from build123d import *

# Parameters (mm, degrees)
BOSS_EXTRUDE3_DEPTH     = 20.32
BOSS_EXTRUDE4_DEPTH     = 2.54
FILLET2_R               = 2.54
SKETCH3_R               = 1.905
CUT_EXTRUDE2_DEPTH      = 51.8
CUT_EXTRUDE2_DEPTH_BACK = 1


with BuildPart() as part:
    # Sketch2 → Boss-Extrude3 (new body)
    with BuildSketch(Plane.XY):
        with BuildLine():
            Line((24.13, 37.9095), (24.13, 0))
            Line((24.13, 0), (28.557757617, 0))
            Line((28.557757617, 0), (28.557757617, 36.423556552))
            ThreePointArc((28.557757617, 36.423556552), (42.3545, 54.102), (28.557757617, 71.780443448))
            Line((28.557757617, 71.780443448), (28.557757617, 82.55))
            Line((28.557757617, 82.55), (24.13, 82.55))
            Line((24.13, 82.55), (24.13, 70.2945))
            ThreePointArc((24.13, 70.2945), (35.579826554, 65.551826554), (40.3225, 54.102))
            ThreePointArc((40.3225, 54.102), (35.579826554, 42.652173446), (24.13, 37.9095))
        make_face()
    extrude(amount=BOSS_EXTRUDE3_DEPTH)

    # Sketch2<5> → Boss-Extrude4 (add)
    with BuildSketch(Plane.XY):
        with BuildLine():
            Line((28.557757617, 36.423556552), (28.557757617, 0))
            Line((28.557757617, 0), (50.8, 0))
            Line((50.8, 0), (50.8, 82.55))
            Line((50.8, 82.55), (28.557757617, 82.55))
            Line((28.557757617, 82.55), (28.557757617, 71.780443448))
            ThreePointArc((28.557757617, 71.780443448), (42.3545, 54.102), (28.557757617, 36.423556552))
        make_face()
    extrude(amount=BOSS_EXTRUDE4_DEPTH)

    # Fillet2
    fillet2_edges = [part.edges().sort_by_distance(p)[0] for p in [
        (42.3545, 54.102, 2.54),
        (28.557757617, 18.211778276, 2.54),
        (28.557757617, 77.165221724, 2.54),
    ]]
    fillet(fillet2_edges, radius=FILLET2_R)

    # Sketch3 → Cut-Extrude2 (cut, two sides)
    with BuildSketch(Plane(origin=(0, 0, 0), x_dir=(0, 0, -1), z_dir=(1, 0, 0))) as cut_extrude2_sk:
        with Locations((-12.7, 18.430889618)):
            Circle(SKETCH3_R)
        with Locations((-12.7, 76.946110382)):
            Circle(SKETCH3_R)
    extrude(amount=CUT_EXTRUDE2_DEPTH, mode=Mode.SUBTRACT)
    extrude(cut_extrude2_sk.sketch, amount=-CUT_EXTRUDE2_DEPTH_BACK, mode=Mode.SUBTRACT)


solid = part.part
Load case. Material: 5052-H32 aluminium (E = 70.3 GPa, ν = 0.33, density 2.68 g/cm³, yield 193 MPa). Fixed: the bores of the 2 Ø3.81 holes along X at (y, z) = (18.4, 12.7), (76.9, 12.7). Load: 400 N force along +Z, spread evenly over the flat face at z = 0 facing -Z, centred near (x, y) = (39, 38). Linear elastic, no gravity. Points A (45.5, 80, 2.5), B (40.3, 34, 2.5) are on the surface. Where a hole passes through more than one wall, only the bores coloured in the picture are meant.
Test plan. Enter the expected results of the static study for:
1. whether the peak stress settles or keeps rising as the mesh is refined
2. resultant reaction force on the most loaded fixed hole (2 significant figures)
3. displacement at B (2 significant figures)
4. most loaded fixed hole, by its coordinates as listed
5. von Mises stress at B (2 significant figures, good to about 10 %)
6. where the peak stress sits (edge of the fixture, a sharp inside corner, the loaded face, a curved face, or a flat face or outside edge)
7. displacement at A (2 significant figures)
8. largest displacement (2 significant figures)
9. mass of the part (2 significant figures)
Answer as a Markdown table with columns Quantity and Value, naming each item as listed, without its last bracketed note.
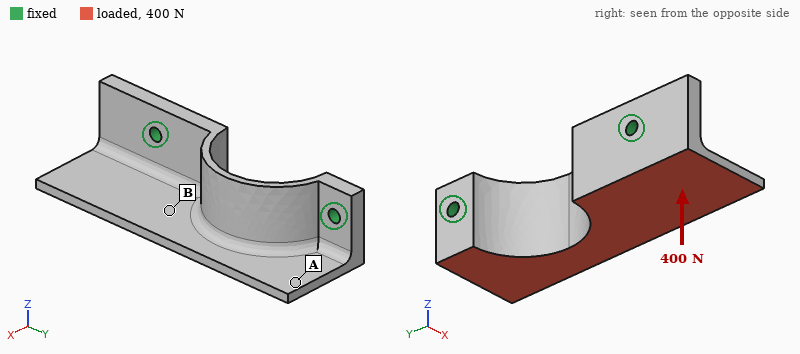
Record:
| Quantity | Value |
|---|---|
| whether the peak stress settles or keeps rising as the mesh is refined | keeps rising |
| resultant reaction force on the most loaded fixed hole | 240 N |
| displacement at B | 0.037 mm |
| most loaded fixed hole, by its coordinates as listed | (18.4, 12.7) |
| von Mises stress at B | 13 MPa |
| where the peak stress sits | edge of the fixture |
| displacement at A | 0.041 mm |
| largest displacement | 0.10 mm |
| mass of the part | 27 g |
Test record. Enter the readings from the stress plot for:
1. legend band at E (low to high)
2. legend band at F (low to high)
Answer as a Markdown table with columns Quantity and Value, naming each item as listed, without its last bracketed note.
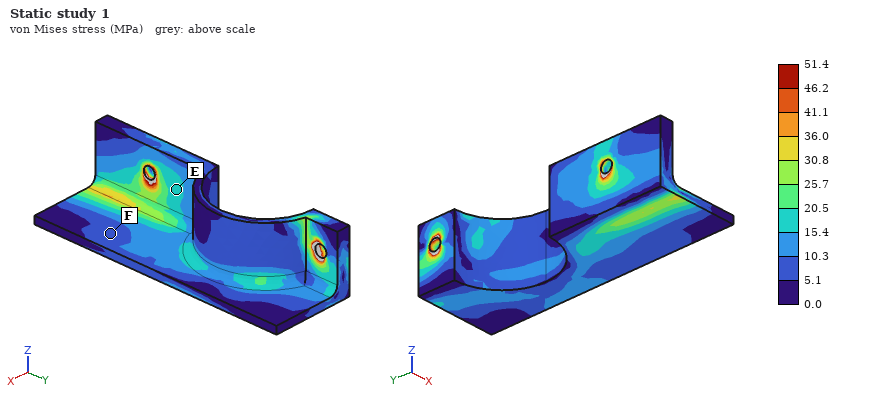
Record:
| Quantity | Value |
|---|---|
| legend band at E | 15.4 to 20.5 MPa |
| legend band at F | 5.1 to 10.3 MPa |
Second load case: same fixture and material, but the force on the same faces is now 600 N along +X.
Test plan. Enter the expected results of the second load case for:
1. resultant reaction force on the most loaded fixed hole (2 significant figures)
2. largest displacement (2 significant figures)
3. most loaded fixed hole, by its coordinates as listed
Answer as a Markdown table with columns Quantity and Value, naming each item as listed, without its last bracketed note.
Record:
| Quantity | Value |
|---|---|
| resultant reaction force on the most loaded fixed hole | 400 N |
| largest displacement | 71 µm |
| most loaded fixed hole, by its coordinates as listed | (18.4, 12.7) |
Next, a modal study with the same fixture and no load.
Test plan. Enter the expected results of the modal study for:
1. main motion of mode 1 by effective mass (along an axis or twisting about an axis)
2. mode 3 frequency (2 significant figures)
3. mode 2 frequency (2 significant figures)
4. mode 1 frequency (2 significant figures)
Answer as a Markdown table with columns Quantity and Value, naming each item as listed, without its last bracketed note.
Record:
| Quantity | Value |
|---|---|
| main motion of mode 1 by effective mass | along Z |
| mode 3 frequency | 6500 Hz |
| mode 2 frequency | 4700 Hz |
| mode 1 frequency | 3600 Hz |
